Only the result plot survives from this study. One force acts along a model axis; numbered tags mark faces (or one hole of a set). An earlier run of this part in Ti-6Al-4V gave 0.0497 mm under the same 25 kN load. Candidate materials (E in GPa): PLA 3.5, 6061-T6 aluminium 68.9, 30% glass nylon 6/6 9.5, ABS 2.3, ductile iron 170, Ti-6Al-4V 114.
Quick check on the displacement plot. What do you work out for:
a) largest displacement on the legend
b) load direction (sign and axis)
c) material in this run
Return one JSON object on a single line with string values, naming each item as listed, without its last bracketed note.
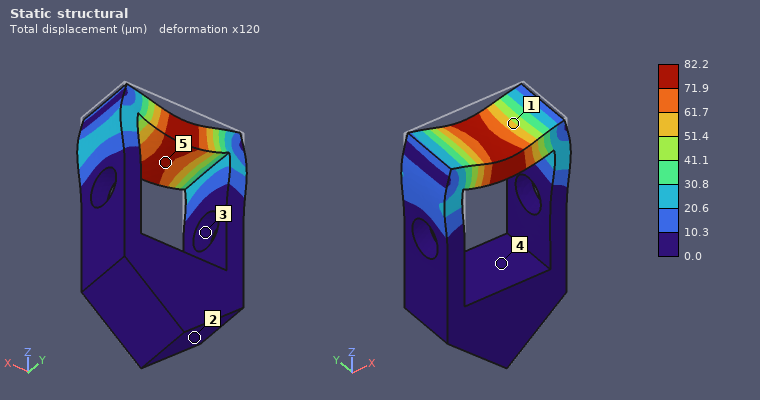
{"largest displacement on the legend": "82.2 µm", "load direction": "-Z", "material in this run": "6061-T6 aluminium"}
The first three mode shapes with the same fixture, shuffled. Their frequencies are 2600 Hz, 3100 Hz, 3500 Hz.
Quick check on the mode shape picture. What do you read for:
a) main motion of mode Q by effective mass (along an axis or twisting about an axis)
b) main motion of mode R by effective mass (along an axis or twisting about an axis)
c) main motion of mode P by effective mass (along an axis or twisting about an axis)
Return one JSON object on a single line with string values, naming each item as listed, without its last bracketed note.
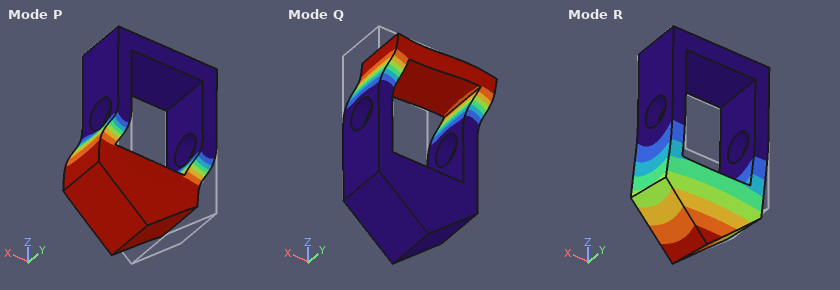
{"main motion of mode Q by effective mass": "along X", "main motion of mode R by effective mass": "along Y", "main motion of mode P by effective mass": "along X"}
